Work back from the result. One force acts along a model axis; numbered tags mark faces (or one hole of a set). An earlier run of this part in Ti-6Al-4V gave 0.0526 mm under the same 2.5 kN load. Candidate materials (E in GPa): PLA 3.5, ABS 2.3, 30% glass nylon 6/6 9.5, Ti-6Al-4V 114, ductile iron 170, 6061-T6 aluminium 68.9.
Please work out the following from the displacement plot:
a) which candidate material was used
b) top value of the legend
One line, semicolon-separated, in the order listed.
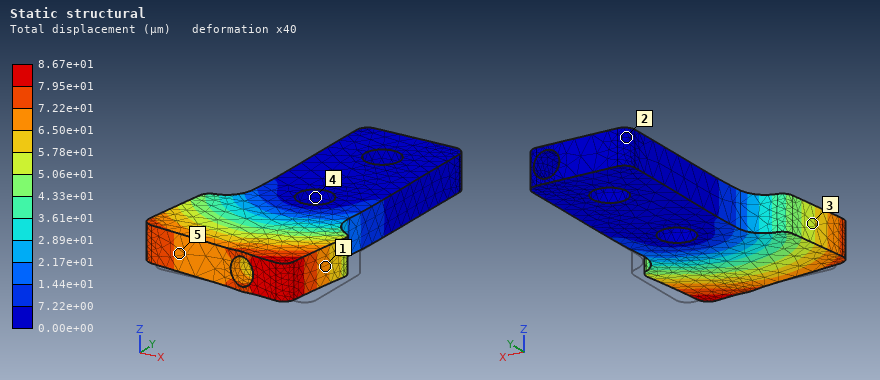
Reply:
6061-T6 aluminium; 8.67e+01 µm
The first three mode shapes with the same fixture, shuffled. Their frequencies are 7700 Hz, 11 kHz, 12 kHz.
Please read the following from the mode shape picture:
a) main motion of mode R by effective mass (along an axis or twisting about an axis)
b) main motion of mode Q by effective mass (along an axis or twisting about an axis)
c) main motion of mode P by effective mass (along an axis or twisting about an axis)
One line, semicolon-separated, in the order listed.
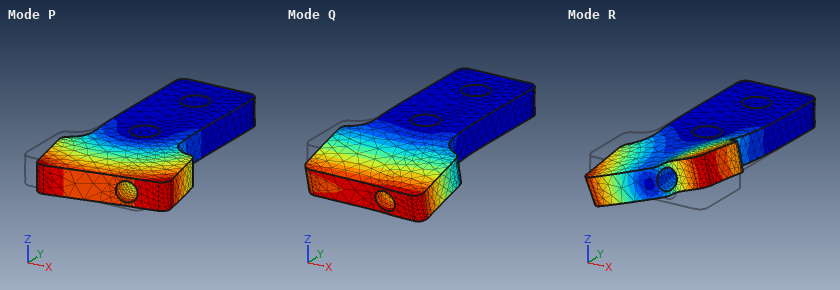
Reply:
twisting about Y; along Z; along X
